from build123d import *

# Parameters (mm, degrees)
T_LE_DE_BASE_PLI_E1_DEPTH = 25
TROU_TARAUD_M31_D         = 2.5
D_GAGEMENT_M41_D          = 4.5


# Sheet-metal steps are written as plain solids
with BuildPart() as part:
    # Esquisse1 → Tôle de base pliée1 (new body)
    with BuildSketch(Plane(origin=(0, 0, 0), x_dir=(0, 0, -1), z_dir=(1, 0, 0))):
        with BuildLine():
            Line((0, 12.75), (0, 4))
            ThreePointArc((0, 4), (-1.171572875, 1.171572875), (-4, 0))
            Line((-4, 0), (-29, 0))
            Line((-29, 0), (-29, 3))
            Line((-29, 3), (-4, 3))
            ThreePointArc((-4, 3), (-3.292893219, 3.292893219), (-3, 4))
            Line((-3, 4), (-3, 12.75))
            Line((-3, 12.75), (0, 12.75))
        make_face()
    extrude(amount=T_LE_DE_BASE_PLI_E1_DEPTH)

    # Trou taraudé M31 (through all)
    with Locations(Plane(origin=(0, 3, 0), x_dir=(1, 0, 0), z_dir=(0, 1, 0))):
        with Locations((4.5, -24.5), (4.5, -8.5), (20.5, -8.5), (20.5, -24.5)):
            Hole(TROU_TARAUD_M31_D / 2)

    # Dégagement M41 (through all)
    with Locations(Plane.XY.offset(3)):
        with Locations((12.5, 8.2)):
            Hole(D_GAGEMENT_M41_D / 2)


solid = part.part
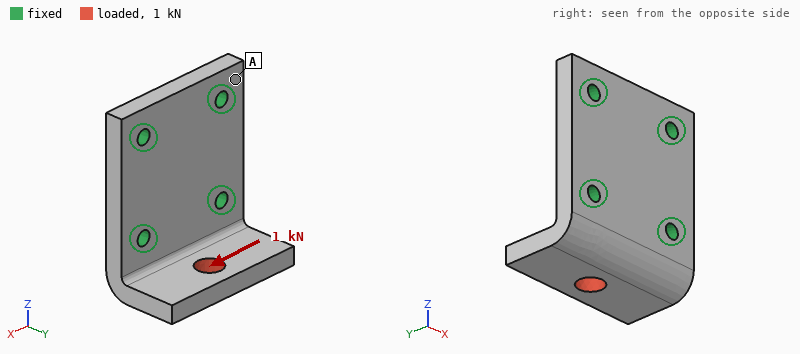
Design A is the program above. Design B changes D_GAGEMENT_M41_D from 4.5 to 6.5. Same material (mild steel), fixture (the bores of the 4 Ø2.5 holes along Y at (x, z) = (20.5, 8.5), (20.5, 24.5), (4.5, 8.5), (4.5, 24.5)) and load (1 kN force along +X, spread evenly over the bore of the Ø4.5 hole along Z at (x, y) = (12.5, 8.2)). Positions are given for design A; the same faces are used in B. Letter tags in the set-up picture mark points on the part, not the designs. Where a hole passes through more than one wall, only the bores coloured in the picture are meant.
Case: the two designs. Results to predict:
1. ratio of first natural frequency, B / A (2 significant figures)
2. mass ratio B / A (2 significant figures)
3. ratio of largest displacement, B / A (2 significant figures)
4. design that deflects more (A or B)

1.0
0.98
1.1
B
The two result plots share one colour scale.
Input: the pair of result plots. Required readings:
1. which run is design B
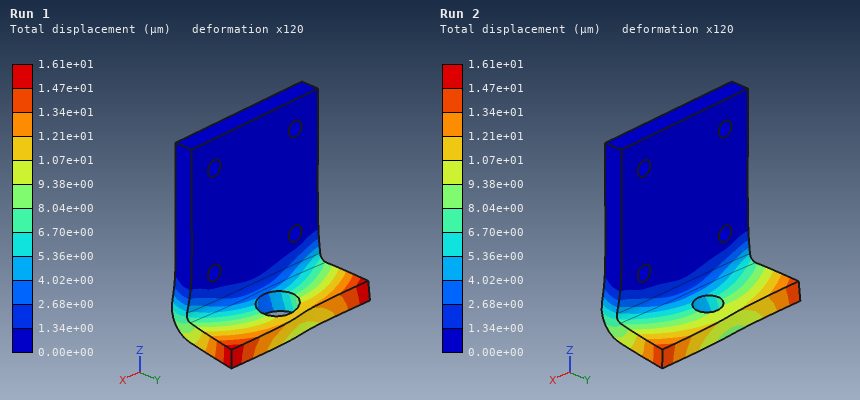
Run 1
